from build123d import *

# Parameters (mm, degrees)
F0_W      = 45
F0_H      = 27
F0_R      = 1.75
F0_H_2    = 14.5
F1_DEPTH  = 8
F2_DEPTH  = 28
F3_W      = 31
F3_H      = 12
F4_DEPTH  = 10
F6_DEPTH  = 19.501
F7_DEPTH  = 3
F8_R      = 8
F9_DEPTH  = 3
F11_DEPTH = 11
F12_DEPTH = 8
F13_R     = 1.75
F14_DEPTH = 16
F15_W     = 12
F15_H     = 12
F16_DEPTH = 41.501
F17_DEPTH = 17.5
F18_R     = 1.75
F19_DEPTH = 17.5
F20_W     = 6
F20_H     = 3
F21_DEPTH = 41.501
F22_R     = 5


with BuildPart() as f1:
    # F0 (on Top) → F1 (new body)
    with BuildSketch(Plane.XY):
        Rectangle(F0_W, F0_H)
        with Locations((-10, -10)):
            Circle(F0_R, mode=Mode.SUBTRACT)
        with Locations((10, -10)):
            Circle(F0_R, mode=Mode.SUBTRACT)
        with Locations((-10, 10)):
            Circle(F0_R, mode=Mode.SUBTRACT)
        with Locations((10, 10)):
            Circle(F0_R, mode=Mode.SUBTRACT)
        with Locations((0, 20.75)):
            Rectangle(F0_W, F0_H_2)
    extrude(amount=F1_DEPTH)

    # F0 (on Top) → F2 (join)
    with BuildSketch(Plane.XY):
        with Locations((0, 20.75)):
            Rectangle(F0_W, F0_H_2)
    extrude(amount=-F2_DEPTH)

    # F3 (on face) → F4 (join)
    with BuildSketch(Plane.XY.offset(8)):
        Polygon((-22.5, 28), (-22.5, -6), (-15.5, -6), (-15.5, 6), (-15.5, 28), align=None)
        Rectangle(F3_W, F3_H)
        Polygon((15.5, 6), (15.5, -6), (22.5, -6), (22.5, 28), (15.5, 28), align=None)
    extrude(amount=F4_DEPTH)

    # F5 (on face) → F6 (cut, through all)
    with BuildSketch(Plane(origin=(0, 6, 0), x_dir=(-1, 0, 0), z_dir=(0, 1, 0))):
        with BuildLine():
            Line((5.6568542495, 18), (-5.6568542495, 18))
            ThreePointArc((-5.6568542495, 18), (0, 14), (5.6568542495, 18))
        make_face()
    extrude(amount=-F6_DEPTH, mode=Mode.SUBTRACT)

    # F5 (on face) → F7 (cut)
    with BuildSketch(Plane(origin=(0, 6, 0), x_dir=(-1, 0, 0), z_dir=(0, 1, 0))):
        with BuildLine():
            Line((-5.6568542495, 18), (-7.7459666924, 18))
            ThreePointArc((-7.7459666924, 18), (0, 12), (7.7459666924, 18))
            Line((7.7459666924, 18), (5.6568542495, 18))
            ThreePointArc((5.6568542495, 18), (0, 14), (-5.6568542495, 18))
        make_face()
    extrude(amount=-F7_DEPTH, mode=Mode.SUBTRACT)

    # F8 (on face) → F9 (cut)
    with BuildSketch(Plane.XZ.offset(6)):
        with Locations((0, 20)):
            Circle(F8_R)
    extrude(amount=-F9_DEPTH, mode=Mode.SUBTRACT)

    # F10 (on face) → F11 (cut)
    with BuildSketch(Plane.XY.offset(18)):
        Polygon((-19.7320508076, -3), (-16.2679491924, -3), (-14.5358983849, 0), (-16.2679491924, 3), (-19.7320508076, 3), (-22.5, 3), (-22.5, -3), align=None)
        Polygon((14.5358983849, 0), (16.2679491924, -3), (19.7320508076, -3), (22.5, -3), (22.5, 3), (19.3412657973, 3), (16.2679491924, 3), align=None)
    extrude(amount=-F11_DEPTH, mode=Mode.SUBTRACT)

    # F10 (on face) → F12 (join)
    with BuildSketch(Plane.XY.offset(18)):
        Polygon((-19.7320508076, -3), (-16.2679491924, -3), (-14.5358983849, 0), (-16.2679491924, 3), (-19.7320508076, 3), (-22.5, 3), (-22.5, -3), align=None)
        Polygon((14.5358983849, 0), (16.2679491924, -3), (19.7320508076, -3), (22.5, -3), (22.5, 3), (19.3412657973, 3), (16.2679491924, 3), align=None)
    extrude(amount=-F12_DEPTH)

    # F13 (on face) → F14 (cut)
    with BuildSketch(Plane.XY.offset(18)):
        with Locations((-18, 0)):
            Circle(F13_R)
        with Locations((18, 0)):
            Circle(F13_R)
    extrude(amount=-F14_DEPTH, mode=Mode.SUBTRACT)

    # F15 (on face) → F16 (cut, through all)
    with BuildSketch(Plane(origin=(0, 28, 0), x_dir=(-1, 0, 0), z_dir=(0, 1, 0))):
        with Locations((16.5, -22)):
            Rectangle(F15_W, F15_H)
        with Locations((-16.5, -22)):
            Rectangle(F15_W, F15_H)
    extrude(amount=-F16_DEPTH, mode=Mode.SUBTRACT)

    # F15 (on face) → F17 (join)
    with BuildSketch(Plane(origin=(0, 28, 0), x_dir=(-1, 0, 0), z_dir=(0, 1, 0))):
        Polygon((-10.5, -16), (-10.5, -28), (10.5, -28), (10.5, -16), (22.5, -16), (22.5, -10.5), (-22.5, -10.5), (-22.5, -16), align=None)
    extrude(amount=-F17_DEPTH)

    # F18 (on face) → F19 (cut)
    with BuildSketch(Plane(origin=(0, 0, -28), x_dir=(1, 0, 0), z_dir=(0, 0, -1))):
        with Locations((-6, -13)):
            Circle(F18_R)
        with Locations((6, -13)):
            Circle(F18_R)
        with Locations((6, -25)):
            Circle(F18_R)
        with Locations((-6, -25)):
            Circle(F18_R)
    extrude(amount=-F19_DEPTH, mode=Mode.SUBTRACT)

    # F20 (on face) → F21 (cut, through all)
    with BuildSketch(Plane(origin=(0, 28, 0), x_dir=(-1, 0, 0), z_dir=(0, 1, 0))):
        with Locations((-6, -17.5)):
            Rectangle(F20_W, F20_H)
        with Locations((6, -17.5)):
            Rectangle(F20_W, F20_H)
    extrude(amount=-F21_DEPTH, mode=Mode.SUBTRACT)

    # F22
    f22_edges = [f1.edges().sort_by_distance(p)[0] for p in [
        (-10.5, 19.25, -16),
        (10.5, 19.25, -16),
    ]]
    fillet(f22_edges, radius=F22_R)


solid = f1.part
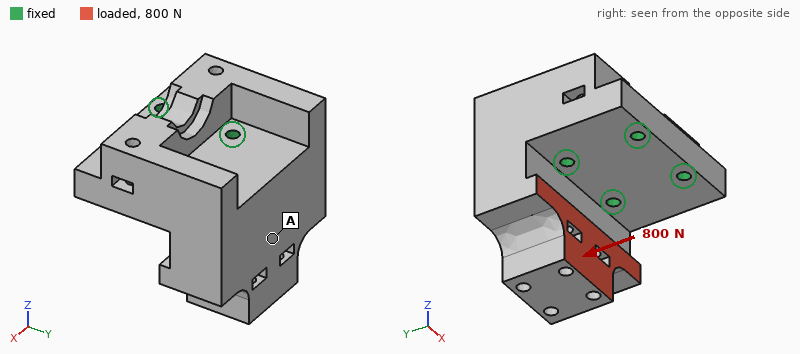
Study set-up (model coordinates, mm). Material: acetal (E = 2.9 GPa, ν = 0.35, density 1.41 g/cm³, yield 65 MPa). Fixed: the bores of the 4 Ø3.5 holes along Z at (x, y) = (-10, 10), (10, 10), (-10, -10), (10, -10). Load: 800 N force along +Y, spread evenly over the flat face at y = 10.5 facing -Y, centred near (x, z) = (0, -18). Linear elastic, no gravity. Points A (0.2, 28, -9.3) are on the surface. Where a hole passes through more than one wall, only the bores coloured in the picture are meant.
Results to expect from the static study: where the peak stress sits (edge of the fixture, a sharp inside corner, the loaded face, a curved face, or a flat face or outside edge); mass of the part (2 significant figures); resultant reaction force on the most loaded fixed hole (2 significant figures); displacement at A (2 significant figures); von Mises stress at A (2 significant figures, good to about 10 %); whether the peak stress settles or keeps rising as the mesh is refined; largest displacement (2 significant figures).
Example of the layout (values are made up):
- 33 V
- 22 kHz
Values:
- edge of the fixture
- 52 g
- 520 N
- 0.36 mm
- 5.0 MPa
- keeps rising
- 0.70 mm
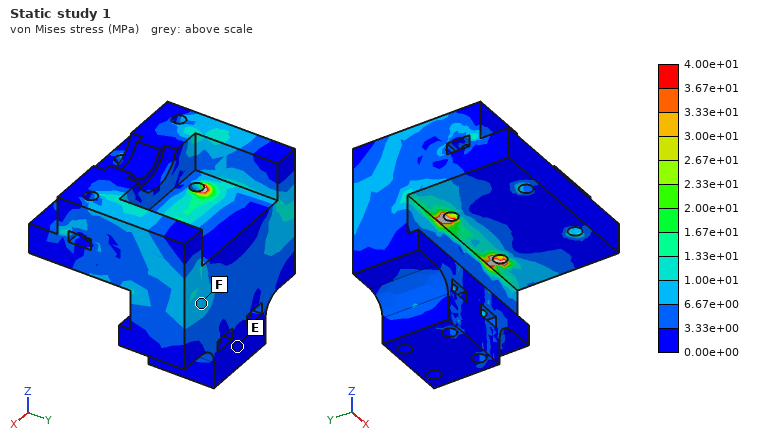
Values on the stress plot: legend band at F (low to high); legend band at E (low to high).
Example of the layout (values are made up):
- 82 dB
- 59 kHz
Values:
- 6.67e+00 to 1.00e+01 MPa
- 0.00e+00 to 3.33e+00 MPa
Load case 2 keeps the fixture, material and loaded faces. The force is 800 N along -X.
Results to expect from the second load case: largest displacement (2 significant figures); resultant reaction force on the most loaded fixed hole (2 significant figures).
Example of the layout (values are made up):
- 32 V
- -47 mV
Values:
- 0.32 mm
- 780 N
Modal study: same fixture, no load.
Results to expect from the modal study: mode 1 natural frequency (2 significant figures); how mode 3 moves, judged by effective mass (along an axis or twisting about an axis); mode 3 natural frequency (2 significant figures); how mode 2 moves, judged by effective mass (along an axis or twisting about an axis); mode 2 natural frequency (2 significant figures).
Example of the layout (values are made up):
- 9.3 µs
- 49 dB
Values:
- 1700 Hz
- along X
- 4200 Hz
- along X
- 2600 Hz
